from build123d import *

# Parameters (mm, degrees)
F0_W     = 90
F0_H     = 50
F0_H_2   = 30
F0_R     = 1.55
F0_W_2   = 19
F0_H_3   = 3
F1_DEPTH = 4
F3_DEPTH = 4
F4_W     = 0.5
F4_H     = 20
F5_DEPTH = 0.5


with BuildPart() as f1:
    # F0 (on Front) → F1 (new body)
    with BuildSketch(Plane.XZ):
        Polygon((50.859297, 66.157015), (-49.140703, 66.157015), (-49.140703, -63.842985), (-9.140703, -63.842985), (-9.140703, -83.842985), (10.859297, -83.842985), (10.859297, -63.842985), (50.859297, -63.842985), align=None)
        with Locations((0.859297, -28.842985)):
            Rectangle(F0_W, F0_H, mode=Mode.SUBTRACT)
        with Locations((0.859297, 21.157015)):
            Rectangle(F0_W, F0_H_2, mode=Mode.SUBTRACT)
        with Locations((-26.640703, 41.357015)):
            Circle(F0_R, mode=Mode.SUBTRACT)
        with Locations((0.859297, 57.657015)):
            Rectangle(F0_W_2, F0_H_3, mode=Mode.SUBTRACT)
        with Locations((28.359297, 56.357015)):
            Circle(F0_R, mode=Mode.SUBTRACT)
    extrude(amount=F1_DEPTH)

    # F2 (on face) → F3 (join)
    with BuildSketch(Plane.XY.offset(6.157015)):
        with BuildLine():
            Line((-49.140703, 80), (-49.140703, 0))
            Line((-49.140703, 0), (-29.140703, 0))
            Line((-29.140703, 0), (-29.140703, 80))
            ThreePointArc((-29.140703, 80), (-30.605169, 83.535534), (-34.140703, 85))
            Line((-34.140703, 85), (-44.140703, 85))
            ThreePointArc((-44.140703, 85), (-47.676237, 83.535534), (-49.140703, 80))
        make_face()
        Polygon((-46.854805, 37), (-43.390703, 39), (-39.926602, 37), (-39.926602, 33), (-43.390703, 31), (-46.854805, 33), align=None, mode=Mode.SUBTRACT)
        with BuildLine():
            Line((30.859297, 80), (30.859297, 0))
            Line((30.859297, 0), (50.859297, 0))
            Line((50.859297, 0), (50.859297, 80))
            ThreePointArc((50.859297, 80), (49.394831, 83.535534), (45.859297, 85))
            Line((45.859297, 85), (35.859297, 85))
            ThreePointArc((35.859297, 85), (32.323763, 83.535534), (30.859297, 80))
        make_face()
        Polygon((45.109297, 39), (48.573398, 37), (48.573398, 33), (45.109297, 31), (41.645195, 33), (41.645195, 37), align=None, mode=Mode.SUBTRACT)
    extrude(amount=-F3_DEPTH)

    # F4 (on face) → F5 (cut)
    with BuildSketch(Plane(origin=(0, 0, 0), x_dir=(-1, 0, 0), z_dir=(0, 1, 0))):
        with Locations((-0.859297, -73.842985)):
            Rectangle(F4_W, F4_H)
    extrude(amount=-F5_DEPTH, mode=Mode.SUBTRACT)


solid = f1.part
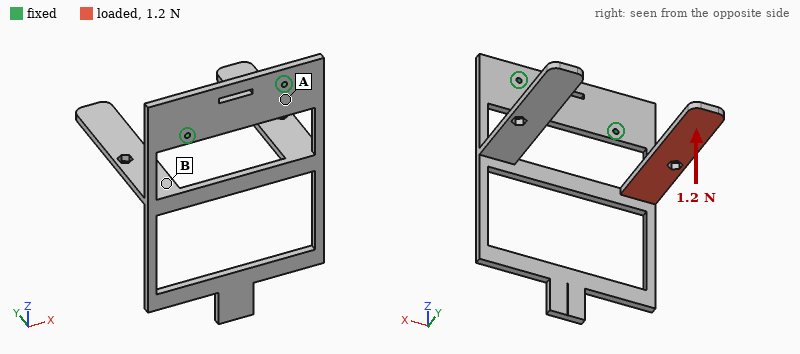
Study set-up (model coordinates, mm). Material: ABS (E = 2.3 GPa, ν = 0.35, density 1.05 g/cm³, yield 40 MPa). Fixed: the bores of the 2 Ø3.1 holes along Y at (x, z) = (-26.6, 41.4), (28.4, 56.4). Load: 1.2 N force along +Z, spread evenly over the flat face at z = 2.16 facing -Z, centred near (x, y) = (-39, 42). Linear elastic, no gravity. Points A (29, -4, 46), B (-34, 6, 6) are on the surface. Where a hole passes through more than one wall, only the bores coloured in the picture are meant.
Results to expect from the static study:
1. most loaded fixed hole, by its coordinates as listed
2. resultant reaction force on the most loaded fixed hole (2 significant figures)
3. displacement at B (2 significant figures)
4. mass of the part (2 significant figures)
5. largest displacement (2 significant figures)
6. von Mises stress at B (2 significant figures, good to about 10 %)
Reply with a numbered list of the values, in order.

1. (-26.6, 41.4)
2. 1.4 N
3. 0.40 mm
4. 40 g
5. 2.3 mm
6. 0.73 MPa
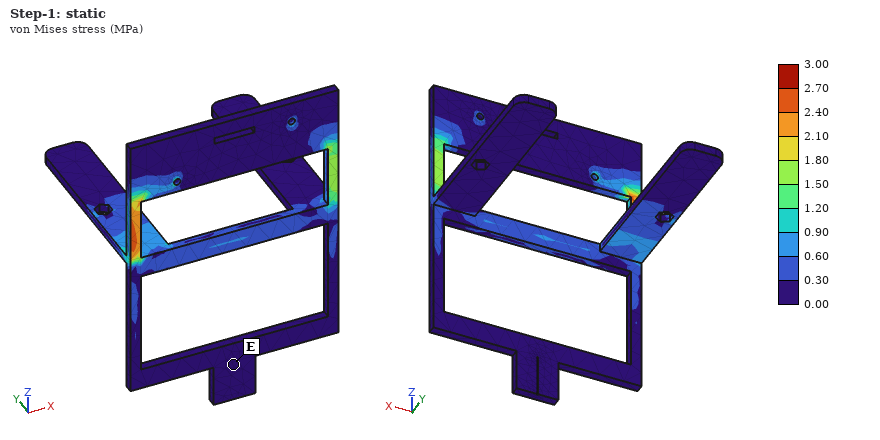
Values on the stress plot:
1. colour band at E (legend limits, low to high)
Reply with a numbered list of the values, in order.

1. 0.00 to 0.30 MPa
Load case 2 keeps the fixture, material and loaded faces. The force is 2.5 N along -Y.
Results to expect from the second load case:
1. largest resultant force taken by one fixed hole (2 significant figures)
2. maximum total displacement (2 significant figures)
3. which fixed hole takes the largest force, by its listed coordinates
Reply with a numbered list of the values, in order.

1. 2.3 N
2. 2.1 mm
3. (-26.6, 41.4)
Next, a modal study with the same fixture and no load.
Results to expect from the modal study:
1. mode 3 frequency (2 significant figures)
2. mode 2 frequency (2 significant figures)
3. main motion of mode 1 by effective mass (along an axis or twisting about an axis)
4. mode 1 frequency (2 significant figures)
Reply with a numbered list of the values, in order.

1. 85 Hz
2. 67 Hz
3. along Y
4. 27 Hz
